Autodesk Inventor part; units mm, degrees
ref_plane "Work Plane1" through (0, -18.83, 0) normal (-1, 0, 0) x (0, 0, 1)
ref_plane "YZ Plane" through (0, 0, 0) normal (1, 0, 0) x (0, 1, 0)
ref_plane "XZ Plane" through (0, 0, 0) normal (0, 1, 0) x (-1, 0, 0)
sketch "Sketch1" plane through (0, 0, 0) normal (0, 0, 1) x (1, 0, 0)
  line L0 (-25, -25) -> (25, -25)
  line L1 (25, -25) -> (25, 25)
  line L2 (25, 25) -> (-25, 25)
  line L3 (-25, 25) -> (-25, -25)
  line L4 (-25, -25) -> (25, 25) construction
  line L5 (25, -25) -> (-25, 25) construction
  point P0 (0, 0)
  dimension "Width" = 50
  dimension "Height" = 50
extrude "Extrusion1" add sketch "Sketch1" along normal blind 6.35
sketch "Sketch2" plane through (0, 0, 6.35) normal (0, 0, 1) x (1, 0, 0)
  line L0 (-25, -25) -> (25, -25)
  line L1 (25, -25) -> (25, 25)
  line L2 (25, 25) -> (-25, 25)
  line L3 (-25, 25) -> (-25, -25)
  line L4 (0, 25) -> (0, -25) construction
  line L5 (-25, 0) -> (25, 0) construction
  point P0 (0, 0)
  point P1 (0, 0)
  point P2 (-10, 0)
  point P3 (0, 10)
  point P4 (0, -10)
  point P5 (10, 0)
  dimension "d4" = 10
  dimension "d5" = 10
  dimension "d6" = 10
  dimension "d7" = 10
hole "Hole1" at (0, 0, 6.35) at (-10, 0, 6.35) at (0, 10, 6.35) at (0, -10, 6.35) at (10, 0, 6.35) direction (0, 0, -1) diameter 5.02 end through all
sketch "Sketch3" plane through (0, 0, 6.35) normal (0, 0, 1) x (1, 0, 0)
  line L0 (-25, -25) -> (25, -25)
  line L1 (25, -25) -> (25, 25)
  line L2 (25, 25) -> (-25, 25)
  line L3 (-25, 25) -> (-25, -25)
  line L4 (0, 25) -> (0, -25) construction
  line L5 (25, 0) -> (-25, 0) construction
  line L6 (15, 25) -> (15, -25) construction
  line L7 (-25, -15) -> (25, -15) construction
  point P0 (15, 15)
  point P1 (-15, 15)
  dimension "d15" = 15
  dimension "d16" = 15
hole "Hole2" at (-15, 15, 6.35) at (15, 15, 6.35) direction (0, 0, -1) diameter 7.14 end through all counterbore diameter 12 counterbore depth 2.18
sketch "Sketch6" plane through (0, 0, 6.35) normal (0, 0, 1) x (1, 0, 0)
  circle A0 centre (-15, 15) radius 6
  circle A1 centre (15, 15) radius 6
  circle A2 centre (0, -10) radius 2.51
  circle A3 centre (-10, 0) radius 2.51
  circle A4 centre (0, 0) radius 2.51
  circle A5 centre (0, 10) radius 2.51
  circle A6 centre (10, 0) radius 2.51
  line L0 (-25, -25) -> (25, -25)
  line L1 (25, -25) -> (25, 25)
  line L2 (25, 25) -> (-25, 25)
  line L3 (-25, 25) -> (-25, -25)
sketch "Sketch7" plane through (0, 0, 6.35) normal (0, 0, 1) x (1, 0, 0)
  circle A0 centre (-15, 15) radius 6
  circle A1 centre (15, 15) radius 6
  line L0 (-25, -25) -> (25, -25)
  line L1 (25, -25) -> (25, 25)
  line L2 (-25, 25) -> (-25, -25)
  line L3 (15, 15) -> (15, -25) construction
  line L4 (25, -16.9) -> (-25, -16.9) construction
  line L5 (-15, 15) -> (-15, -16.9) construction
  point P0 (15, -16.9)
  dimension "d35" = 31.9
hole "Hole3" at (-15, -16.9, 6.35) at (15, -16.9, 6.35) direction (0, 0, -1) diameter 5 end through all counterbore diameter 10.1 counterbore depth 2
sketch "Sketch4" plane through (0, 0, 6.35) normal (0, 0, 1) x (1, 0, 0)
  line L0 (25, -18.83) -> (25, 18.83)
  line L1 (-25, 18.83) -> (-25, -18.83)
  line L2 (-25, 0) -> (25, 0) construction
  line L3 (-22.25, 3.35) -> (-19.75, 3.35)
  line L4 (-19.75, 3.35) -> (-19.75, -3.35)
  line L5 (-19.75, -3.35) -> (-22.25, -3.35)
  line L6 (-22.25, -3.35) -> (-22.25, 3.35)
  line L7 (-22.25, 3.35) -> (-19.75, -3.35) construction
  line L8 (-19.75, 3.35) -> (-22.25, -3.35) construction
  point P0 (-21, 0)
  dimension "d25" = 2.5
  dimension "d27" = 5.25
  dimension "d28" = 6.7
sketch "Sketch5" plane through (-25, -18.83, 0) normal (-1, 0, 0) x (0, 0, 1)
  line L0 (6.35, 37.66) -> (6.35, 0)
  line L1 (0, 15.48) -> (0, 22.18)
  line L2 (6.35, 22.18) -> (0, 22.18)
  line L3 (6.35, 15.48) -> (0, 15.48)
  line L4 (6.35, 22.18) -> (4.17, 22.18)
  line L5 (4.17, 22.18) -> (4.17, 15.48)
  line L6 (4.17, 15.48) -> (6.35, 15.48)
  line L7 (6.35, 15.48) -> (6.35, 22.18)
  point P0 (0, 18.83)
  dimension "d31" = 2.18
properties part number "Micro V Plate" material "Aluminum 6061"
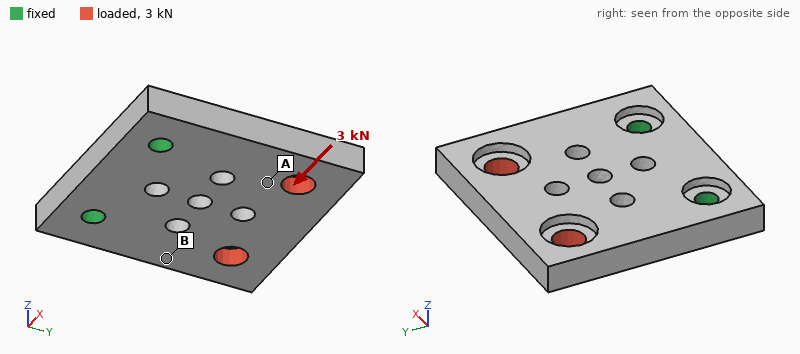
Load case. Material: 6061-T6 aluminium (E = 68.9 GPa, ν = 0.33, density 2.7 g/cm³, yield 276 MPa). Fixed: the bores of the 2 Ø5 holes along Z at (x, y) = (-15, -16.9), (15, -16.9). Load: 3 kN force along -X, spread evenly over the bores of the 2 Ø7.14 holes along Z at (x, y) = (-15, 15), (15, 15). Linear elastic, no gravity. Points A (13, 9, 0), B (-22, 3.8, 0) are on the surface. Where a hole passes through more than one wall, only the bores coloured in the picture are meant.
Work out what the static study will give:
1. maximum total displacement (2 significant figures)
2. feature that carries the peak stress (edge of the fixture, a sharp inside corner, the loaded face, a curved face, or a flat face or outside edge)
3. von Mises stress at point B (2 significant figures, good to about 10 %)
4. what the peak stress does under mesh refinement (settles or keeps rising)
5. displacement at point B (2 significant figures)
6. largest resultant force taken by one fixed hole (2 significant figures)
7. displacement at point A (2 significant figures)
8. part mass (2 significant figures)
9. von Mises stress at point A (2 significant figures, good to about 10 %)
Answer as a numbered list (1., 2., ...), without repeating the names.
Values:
1. 58 µm
2. edge of the fixture
3. 17 MPa
4. keeps rising
5. 31 µm
6. 3.2 kN
7. 33 µm
8. 38 g
9. 45 MPa
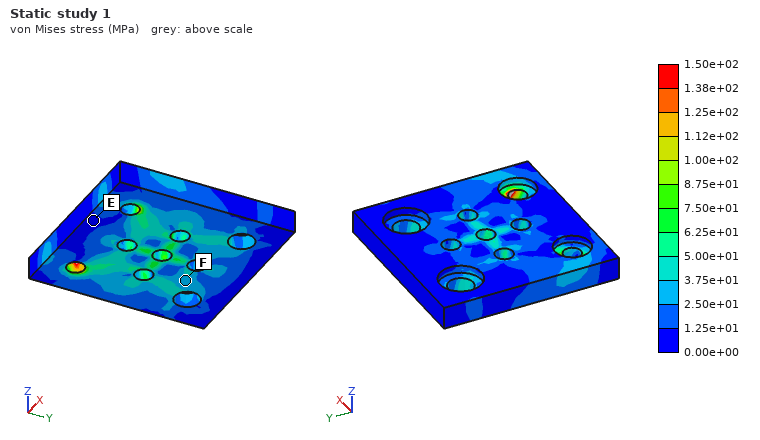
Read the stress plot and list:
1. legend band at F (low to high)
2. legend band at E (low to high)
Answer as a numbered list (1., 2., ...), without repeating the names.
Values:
1. 2.50e+01 to 3.75e+01 MPa
2. 0.00e+00 to 1.25e+01 MPa
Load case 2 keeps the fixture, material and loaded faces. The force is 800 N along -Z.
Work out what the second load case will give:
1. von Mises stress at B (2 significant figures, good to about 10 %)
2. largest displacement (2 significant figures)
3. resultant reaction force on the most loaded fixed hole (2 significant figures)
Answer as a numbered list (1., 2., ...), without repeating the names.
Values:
1. 33 MPa
2. 0.28 mm
3. 410 N
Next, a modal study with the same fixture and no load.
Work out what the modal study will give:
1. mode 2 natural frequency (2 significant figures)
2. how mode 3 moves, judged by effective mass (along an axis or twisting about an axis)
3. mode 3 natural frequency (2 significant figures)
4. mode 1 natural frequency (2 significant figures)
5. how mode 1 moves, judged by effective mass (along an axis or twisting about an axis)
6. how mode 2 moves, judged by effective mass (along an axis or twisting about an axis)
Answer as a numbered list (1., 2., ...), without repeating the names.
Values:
1. 5300 Hz
2. along X
3. 11 kHz
4. 2400 Hz
5. along Z
6. twisting about Y
